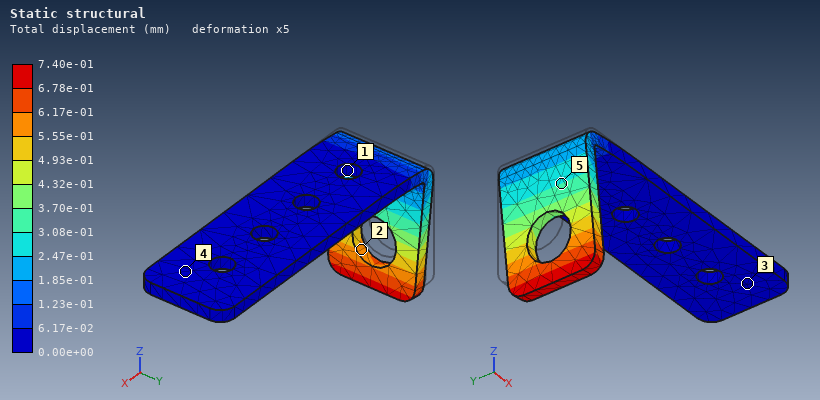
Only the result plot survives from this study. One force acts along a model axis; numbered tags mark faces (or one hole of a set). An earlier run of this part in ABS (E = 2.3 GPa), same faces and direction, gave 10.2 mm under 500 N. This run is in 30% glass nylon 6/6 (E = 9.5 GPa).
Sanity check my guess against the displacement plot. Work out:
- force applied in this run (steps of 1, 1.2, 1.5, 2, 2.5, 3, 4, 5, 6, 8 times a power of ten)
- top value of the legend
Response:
150 N
7.40e-01 mm
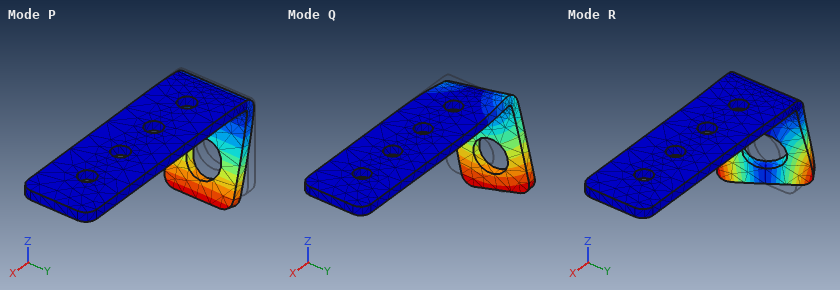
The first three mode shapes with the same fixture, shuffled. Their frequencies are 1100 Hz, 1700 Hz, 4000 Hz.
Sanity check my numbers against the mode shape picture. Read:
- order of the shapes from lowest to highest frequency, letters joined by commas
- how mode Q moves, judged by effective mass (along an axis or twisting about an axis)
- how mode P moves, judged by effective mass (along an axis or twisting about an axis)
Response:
P, Q, R
along Y
along X
